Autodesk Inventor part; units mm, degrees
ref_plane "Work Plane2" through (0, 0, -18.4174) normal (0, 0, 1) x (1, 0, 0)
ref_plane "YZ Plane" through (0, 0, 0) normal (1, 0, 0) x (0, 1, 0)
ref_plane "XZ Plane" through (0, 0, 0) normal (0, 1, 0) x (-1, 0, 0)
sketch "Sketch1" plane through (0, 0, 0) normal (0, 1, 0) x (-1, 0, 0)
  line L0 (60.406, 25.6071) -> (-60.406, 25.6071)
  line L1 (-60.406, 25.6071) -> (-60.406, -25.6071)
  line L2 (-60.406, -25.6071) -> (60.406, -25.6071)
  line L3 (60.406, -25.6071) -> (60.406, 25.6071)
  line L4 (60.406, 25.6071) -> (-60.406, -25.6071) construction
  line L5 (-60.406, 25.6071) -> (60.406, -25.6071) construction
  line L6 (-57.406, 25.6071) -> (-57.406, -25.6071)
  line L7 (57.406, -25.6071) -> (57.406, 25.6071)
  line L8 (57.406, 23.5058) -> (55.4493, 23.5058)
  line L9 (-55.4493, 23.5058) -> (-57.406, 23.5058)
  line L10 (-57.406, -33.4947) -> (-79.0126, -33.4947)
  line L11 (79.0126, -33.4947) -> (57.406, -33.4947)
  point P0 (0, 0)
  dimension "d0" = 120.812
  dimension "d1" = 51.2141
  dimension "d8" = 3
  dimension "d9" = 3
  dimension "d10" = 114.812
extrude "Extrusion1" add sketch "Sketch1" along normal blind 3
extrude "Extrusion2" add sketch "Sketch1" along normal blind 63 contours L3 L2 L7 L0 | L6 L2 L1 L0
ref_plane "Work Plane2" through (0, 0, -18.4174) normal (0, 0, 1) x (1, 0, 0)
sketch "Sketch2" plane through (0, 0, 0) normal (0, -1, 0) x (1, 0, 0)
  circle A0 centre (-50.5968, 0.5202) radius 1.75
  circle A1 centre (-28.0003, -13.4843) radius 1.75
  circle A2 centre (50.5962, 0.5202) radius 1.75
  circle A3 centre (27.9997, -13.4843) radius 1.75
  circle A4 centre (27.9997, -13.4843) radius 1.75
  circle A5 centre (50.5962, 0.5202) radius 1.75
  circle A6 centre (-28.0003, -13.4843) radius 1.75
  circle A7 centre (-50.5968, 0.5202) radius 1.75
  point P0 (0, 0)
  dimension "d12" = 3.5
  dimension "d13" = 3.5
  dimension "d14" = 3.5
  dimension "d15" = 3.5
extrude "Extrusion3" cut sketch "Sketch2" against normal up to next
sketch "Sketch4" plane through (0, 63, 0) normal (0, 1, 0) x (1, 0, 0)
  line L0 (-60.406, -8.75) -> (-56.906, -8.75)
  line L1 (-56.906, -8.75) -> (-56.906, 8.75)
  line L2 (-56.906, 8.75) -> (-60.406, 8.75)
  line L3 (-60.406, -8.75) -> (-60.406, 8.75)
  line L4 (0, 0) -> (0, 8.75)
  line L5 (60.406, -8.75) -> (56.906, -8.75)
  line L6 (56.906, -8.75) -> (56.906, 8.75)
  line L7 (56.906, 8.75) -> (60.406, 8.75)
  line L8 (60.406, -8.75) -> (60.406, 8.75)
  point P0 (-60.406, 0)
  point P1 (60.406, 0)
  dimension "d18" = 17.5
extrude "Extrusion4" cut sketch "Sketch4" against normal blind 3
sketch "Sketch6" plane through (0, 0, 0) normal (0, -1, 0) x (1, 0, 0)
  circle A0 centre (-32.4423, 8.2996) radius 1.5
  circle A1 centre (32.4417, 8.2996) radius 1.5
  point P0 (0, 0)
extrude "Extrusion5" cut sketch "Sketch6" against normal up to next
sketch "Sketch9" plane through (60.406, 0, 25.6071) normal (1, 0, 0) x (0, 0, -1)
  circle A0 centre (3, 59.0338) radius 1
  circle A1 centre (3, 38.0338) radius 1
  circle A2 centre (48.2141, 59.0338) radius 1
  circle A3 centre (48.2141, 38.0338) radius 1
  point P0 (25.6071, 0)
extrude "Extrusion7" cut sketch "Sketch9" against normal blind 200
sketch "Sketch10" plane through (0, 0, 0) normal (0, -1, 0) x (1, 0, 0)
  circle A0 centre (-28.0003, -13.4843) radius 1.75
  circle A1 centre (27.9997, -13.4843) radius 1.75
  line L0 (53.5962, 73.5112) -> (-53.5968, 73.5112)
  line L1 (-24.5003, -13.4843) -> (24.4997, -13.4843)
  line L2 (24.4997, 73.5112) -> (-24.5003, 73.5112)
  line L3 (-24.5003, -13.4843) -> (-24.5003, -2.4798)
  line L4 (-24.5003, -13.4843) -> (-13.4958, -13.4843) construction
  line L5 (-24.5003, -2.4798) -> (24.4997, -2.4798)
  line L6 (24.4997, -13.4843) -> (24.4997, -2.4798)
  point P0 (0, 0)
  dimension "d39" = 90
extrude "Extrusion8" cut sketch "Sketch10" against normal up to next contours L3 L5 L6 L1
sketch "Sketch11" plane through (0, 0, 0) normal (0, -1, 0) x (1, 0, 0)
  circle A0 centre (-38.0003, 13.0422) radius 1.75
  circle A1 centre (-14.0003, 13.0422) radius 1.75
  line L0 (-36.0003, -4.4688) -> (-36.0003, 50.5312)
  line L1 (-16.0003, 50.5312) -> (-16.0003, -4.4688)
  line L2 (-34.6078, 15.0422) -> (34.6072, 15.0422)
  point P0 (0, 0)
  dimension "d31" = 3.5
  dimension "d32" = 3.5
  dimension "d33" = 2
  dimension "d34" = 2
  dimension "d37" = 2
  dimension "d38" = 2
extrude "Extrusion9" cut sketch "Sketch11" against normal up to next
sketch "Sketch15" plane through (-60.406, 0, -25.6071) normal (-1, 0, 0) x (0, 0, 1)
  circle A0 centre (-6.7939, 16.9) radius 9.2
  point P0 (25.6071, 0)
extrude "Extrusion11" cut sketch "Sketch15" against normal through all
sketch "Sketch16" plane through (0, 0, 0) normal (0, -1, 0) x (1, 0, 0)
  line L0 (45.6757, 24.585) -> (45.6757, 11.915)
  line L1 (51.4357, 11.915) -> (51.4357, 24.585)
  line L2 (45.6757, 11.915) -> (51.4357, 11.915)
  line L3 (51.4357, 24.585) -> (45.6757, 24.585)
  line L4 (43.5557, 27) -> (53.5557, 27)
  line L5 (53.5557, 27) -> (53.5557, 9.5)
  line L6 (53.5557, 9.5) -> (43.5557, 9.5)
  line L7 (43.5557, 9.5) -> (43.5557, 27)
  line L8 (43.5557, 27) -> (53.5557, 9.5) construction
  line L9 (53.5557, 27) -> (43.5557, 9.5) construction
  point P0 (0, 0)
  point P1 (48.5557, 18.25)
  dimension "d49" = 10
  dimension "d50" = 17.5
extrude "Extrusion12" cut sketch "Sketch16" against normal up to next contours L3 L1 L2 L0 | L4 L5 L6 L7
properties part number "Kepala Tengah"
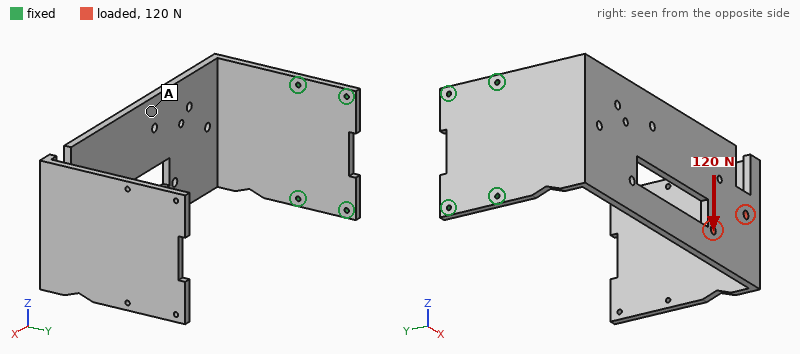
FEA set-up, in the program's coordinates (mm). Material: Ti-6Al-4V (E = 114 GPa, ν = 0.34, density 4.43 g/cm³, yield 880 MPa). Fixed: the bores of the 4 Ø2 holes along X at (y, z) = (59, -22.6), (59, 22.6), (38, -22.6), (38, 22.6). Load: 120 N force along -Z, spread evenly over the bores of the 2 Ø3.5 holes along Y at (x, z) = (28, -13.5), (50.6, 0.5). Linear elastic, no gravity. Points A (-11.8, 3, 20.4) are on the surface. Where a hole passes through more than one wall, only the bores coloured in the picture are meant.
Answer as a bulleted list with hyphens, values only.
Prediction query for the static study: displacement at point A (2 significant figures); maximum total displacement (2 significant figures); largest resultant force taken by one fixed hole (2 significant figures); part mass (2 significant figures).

- 0.64 mm
- 1.7 mm
- 330 N
- 150 g
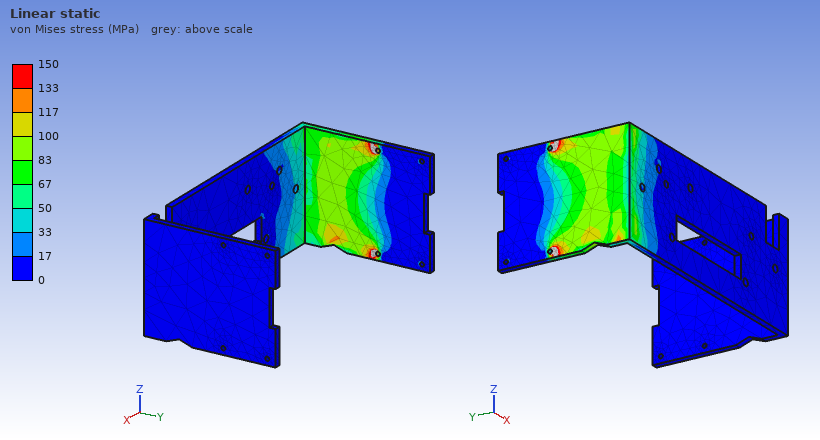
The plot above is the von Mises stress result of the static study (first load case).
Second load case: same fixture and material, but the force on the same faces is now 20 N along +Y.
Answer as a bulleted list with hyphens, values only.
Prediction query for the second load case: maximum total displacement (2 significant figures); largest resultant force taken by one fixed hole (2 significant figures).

- 1.6 mm
- 28 N
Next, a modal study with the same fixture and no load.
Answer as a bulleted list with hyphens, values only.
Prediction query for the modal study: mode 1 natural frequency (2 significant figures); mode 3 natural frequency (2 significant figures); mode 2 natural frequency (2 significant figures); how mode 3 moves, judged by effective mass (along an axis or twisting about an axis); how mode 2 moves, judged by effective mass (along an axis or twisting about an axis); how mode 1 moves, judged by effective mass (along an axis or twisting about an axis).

- 68 Hz
- 260 Hz
- 140 Hz
- along X
- along Z
- along Y
